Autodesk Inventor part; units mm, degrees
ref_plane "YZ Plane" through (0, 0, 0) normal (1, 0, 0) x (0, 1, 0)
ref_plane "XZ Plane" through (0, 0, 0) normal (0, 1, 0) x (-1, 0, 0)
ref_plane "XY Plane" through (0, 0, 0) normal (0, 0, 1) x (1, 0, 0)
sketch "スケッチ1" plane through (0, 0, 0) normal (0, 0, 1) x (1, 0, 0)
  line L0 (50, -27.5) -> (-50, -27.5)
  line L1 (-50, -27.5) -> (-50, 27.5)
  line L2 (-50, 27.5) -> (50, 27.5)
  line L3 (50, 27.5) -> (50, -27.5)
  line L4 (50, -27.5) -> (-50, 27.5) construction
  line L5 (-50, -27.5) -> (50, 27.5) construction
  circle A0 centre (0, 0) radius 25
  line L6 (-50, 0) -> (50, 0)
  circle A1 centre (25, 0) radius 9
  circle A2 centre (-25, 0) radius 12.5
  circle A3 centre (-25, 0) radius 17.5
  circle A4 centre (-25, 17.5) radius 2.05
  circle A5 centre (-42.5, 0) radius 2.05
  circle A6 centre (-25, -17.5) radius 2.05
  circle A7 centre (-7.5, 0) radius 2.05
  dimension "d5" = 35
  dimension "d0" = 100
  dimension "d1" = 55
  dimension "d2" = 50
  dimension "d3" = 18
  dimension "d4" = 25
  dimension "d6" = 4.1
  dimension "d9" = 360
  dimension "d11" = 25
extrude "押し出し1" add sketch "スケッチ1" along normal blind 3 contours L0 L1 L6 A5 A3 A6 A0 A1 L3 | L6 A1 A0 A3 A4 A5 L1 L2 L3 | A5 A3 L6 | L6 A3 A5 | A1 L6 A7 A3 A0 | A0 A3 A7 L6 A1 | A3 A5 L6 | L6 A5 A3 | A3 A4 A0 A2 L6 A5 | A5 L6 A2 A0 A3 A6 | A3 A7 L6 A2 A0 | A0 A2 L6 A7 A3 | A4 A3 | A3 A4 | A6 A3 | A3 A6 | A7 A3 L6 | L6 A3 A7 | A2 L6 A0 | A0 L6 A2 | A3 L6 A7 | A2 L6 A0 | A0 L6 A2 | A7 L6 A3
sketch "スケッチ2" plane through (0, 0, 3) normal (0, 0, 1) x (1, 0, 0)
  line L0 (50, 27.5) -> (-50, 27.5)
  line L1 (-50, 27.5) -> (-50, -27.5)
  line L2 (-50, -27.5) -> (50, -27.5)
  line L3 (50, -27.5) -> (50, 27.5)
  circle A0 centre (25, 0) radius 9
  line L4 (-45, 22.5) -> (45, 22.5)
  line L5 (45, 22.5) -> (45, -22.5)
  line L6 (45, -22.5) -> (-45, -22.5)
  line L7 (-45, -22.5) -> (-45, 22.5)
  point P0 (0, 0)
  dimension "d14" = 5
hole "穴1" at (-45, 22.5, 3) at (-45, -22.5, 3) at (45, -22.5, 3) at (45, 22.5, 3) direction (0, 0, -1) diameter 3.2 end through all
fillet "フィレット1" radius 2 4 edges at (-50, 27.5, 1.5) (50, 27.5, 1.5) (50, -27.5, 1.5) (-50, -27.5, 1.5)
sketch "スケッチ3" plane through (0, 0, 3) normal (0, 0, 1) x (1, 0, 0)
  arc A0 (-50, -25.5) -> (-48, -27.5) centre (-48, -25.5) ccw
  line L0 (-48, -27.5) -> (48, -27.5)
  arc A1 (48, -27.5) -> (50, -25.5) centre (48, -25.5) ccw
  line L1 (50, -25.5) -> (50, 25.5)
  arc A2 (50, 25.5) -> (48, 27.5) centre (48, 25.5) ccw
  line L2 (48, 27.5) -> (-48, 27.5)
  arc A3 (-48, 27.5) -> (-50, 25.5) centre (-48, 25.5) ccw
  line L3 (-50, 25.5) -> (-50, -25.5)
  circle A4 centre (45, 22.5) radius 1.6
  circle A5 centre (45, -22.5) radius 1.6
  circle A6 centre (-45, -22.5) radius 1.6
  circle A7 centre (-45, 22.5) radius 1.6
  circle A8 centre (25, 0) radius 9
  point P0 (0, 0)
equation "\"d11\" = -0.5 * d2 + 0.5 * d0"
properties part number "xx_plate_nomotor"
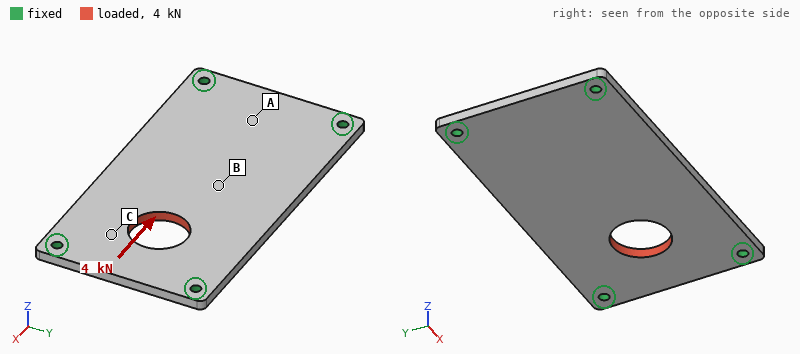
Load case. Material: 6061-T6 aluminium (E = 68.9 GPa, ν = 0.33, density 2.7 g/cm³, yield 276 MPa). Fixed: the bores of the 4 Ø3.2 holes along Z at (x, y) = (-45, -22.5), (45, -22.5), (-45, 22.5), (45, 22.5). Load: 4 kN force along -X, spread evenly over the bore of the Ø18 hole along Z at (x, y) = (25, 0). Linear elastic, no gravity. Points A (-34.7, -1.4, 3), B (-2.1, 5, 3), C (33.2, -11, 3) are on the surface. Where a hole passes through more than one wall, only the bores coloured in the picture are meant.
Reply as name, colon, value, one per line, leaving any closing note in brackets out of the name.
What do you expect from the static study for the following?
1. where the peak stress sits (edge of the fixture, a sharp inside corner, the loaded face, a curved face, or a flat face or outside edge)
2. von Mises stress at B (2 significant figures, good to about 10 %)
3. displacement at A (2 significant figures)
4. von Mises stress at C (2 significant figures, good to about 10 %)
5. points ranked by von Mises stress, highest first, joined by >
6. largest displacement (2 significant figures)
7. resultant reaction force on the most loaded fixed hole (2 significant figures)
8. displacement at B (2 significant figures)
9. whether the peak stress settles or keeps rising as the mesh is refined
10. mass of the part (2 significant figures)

where the peak stress sits: edge of the fixture
von Mises stress at B: 13 MPa
displacement at A: 5.1 µm
von Mises stress at C: 22 MPa
points ranked by von Mises stress, highest first, joined by >: C > B > A
largest displacement: 19 µm
resultant reaction force on the most loaded fixed hole: 1.4 kN
displacement at B: 8.1 µm
whether the peak stress settles or keeps rising as the mesh is refined: keeps rising
mass of the part: 42 g
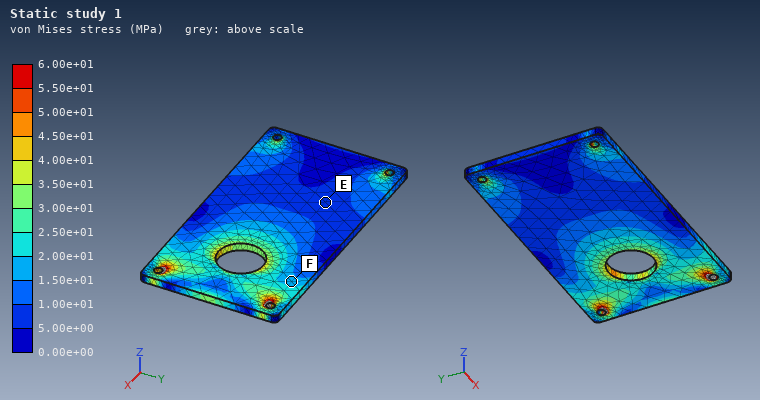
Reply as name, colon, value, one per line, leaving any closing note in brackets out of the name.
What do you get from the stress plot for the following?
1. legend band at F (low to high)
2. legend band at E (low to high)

legend band at F: 1.50e+01 to 2.00e+01 MPa
legend band at E: 5.00e+00 to 1.00e+01 MPa
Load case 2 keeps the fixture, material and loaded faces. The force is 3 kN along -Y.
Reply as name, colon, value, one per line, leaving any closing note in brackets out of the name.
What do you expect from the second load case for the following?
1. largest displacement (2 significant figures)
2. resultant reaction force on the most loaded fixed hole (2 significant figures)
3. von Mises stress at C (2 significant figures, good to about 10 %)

largest displacement: 22 µm
resultant reaction force on the most loaded fixed hole: 1.2 kN
von Mises stress at C: 25 MPa
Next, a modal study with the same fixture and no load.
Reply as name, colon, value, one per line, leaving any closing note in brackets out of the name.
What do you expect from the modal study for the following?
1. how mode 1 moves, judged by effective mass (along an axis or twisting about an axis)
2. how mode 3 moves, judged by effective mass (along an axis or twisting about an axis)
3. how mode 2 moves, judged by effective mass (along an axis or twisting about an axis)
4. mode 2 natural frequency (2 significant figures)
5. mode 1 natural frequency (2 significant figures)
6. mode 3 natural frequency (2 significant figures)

how mode 1 moves, judged by effective mass: along Z
how mode 3 moves, judged by effective mass: twisting about Y
how mode 2 moves, judged by effective mass: twisting about X
mode 2 natural frequency: 2700 Hz
mode 1 natural frequency: 1700 Hz
mode 3 natural frequency: 4600 Hz
